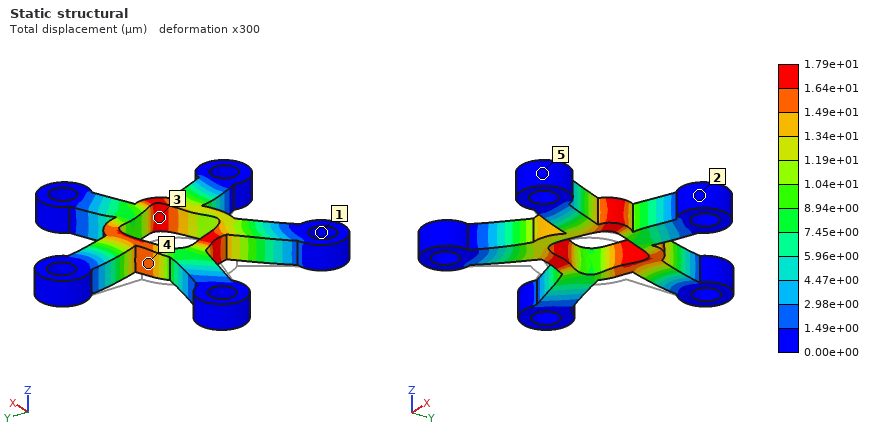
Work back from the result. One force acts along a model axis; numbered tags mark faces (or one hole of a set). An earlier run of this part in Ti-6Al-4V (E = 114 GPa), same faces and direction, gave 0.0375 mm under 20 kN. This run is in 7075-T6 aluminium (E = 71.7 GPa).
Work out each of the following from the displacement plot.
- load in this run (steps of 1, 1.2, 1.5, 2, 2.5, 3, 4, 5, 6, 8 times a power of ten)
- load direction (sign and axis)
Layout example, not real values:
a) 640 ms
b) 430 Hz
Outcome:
a) 6 kN
b) +X
